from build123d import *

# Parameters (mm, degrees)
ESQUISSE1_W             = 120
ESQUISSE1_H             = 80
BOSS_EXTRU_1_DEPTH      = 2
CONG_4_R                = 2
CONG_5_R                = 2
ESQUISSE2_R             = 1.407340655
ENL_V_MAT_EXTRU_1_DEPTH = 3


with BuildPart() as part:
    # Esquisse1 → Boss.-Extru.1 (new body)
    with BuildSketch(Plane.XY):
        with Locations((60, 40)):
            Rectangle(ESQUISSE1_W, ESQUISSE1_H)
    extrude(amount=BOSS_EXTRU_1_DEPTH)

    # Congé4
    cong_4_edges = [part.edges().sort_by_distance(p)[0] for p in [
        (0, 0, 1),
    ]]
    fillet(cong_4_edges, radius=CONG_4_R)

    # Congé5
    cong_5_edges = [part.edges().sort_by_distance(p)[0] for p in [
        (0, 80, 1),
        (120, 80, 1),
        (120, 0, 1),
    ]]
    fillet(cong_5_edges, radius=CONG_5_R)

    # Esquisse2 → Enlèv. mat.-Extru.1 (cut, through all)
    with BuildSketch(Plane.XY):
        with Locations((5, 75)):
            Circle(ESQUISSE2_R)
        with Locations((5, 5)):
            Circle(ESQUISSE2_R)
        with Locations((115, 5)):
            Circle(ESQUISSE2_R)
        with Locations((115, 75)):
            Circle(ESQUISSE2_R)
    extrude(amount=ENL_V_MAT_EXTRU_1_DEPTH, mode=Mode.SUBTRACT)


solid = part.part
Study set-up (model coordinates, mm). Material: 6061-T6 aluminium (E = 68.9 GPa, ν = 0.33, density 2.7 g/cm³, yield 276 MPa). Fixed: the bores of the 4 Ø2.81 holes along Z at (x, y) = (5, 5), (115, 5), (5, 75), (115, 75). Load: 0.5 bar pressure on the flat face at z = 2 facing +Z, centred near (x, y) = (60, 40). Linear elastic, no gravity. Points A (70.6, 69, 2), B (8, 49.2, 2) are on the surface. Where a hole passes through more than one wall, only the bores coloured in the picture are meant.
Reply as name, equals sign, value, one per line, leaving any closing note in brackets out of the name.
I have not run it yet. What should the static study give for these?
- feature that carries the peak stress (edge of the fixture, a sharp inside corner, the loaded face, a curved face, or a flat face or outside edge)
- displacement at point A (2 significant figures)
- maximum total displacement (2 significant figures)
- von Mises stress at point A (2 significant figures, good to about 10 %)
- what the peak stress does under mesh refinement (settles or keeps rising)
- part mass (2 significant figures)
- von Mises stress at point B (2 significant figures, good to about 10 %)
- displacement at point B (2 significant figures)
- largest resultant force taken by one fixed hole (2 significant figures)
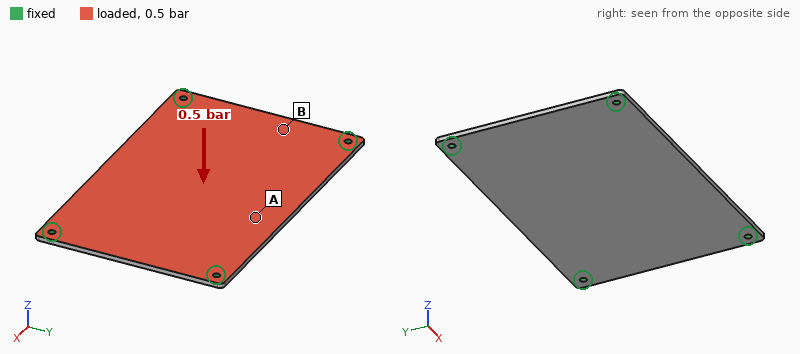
feature that carries the peak stress = edge of the fixture
displacement at point A = 0.60 mm
maximum total displacement = 0.68 mm
von Mises stress at point A = 44 MPa
what the peak stress does under mesh refinement = keeps rising
part mass = 52 g
von Mises stress at point B = 22 MPa
displacement at point B = 0.14 mm
largest resultant force taken by one fixed hole = 120 N
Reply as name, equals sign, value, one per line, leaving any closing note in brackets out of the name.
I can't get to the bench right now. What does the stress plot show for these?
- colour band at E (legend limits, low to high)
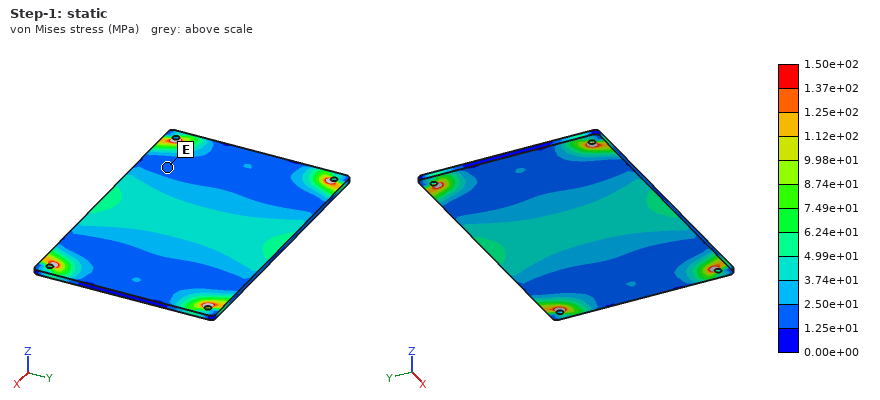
colour band at E = 1.25e+01 to 2.50e+01 MPa
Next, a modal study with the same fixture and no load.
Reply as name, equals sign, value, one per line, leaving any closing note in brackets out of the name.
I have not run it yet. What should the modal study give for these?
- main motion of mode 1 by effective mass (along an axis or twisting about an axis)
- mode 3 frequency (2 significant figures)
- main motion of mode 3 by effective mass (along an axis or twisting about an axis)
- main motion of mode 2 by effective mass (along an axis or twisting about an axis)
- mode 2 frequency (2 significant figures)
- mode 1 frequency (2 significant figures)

main motion of mode 1 by effective mass = along Z
mode 3 frequency = 1700 Hz
main motion of mode 3 by effective mass = twisting about Y
main motion of mode 2 by effective mass = twisting about X
mode 2 frequency = 1100 Hz
mode 1 frequency = 680 Hz
